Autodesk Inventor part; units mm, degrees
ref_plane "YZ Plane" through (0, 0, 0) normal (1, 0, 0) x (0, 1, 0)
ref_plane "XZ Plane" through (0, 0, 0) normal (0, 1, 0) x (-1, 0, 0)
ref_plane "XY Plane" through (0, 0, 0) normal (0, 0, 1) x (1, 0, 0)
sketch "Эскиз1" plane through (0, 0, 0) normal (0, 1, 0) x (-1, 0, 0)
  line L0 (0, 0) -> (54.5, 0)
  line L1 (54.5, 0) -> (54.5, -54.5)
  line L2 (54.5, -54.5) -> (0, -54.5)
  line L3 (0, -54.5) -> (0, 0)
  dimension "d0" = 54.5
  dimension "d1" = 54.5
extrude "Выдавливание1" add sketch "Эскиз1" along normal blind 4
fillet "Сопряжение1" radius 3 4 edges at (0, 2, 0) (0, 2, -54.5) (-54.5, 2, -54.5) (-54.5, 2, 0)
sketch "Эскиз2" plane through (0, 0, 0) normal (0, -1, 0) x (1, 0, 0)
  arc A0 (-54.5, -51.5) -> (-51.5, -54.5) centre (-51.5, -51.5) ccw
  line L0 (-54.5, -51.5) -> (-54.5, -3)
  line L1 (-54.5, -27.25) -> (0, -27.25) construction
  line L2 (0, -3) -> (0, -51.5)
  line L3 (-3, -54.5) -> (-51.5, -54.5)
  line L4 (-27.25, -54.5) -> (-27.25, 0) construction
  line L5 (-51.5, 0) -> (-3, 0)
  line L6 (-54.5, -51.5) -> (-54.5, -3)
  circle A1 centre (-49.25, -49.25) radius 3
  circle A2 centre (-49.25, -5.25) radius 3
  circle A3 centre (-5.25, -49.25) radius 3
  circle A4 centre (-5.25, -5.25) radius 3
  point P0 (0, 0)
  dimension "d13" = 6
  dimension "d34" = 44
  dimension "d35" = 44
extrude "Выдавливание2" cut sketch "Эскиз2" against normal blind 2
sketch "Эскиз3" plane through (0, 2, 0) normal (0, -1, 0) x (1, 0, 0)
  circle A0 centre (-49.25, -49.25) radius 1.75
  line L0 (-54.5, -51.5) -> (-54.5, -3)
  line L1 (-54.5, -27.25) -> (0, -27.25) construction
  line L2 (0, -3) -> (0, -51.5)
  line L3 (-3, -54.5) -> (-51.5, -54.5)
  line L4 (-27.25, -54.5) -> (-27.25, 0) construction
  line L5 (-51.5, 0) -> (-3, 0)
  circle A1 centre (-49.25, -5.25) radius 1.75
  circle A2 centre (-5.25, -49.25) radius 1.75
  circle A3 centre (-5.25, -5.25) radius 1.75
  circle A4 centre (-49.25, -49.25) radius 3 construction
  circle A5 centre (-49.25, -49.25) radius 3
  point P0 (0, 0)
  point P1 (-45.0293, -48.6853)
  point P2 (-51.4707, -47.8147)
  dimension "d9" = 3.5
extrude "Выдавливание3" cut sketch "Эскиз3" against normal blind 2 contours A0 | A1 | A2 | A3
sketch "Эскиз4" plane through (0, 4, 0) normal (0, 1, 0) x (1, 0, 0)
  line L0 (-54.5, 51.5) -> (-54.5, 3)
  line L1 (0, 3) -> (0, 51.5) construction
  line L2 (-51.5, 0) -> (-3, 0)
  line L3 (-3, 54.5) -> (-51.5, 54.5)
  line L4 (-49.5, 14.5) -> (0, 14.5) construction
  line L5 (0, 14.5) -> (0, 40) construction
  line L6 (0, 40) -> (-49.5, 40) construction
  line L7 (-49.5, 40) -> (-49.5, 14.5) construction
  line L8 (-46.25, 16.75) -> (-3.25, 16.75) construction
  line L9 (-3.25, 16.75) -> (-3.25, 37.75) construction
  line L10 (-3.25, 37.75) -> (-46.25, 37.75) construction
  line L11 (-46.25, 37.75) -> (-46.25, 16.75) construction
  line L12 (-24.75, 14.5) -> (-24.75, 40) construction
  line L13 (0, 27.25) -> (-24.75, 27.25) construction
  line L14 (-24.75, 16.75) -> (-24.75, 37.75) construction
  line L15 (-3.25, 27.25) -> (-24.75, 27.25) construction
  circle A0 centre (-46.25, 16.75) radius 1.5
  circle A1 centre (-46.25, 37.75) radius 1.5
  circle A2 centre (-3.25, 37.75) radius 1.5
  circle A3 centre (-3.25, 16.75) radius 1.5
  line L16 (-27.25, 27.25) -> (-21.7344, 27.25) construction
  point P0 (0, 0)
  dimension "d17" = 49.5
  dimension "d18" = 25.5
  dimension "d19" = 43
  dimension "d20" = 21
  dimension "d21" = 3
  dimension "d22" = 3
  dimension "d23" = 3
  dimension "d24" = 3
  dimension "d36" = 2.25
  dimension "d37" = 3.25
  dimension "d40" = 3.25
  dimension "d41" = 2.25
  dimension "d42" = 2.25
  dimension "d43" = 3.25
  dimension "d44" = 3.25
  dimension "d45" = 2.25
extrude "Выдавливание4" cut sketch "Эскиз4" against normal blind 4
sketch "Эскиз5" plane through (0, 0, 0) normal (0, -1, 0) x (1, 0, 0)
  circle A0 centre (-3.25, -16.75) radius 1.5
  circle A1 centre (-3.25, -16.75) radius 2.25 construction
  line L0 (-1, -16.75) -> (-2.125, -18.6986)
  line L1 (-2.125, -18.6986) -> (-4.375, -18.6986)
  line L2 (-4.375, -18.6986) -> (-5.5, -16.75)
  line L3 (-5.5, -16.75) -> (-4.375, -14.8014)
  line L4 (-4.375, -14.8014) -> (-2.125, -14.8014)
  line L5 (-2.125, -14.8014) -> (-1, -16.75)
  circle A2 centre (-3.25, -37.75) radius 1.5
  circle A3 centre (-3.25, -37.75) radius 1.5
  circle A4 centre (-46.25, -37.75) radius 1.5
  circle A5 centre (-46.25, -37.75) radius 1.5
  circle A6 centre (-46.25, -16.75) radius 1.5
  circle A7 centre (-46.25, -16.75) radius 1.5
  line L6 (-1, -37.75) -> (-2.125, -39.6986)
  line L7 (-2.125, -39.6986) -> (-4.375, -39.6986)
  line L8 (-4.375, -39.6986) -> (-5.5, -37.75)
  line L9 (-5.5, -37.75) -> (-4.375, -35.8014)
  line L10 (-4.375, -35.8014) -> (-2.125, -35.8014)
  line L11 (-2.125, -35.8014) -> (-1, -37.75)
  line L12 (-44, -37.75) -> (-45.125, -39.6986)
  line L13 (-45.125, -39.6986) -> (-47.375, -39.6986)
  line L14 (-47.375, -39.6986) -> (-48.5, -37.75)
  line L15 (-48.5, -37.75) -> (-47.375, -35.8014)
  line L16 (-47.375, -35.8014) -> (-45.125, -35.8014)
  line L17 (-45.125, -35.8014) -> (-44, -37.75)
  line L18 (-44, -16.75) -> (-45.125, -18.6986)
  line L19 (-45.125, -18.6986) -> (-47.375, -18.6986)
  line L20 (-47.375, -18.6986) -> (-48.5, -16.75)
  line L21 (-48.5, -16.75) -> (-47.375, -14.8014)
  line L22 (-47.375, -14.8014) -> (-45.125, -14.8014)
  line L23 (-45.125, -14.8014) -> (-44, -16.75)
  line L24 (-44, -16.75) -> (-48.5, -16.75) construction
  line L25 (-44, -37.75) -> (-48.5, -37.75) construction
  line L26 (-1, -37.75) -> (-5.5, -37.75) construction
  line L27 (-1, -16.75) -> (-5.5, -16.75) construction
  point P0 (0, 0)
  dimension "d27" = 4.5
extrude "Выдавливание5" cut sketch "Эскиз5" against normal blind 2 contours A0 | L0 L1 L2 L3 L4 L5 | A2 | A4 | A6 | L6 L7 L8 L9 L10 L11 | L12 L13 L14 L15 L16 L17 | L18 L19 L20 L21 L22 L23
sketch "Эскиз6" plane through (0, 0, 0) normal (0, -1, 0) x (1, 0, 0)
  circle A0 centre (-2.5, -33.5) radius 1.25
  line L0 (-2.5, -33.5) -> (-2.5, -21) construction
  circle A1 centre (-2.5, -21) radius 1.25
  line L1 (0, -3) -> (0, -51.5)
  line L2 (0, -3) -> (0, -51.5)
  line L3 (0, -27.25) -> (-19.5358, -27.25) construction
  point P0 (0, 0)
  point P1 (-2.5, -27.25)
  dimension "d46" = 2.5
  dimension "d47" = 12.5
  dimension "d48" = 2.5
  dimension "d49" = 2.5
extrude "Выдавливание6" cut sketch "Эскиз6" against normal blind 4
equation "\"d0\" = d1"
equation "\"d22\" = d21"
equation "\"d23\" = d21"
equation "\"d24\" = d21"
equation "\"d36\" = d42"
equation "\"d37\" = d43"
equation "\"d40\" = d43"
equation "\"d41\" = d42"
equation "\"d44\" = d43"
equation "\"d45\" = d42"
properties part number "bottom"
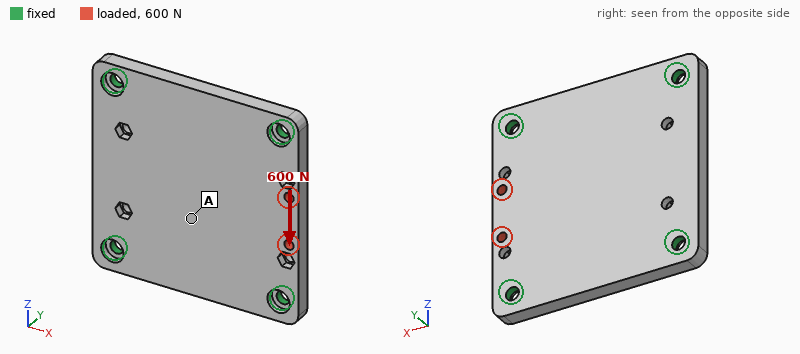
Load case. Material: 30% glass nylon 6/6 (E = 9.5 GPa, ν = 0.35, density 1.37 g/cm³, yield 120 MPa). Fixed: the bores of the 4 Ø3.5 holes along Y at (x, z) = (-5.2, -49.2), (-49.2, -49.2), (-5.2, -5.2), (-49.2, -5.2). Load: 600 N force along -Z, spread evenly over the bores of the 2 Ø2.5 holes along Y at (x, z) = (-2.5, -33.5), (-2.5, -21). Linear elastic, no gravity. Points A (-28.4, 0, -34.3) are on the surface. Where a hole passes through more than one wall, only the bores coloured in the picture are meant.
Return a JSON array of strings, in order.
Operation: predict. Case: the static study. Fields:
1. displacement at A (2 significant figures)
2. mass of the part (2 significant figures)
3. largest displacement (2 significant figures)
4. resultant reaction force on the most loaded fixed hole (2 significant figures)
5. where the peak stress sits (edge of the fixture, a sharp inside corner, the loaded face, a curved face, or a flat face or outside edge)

["4.6 µm", "16 g", "24 µm", "270 N", "a curved face"]
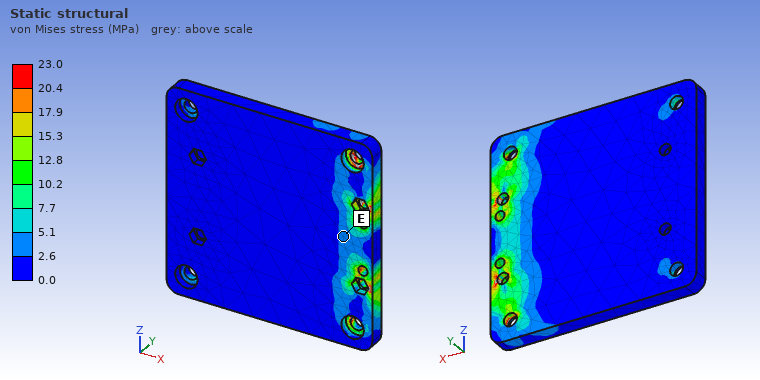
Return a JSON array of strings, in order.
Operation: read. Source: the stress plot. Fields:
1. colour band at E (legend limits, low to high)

["2.6 to 5.1 MPa"]
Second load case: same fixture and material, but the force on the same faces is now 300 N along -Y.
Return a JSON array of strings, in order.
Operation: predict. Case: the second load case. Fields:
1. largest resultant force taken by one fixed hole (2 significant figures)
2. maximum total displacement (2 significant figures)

["230 N", "0.30 mm"]
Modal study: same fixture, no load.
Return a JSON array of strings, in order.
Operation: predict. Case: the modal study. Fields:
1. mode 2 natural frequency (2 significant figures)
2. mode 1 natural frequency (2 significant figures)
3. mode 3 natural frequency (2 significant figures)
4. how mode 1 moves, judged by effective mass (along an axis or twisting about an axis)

["5000 Hz", "3100 Hz", "5000 Hz", "along Y"]
